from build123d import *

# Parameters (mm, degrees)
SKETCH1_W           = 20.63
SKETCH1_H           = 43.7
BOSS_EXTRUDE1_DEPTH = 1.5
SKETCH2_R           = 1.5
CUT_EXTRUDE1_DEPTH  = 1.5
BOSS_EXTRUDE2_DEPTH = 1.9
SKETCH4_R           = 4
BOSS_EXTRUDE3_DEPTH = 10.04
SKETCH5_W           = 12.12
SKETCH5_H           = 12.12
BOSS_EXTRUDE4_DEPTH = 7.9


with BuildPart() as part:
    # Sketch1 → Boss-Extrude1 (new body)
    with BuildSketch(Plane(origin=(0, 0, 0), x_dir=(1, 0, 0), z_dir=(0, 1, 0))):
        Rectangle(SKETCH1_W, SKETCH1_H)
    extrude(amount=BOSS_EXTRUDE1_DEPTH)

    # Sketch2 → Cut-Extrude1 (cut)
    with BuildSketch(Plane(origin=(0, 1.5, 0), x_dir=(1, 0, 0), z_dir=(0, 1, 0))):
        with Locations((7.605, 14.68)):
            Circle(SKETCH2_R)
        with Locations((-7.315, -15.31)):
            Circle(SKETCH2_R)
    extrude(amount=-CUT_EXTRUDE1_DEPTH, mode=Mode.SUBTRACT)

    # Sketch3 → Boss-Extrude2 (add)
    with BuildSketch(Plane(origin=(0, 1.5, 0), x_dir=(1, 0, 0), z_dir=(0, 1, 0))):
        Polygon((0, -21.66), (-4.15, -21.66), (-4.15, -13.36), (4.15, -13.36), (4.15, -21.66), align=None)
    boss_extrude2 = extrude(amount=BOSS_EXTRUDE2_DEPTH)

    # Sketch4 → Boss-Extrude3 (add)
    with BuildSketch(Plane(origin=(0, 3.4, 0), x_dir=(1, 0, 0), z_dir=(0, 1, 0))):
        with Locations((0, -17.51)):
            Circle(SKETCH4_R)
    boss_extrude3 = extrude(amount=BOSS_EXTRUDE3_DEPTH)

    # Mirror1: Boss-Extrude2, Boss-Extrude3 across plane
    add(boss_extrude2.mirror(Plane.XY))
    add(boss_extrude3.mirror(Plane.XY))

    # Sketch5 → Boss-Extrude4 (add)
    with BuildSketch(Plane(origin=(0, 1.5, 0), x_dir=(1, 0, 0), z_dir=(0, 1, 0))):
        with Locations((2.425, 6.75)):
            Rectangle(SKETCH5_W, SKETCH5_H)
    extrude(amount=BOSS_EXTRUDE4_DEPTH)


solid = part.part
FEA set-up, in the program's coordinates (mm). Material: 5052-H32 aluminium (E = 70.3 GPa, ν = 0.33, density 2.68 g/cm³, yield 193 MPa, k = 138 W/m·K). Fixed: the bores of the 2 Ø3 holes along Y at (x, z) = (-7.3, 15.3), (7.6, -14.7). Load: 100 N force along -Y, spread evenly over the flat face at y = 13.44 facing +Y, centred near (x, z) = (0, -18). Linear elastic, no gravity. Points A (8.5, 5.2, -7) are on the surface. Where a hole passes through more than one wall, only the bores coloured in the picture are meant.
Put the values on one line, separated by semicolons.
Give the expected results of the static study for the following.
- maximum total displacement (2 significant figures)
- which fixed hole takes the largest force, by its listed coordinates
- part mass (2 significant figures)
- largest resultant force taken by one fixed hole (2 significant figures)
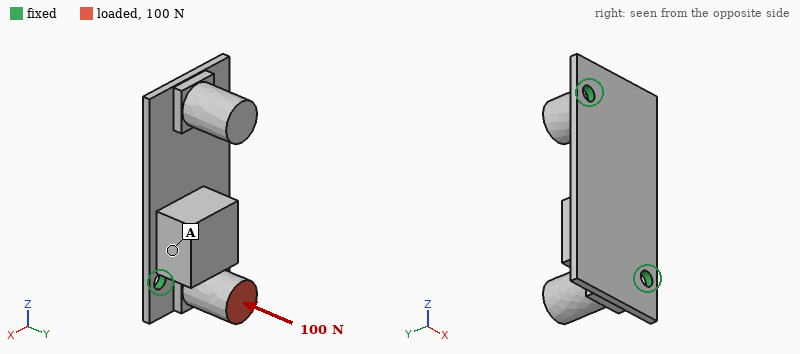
62 µm; (7.6, -14.7); 10 g; 99 N
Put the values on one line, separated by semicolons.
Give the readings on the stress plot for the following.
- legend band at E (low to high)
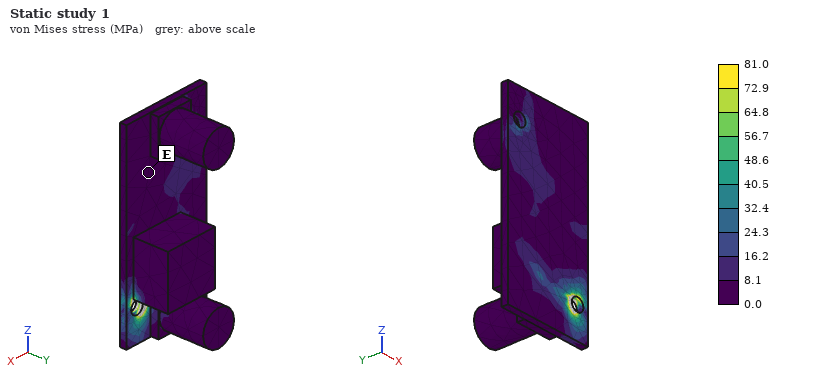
0.0 to 8.1 MPa
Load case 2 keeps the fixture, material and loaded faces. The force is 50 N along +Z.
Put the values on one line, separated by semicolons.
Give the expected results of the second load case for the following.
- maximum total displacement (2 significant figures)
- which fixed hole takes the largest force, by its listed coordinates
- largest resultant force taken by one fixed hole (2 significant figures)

46 µm; (7.6, -14.7); 32 N
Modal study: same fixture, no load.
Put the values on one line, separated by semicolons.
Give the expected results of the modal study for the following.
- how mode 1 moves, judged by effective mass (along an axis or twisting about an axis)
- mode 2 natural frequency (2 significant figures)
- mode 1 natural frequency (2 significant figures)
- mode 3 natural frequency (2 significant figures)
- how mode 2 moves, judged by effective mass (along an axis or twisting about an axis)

along X; 3900 Hz; 3300 Hz; 4900 Hz; along Y
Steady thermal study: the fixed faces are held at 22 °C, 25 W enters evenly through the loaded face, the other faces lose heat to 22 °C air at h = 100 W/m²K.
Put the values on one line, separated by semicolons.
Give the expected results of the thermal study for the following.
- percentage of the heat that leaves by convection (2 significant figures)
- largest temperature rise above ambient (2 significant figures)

20 %; 76 K
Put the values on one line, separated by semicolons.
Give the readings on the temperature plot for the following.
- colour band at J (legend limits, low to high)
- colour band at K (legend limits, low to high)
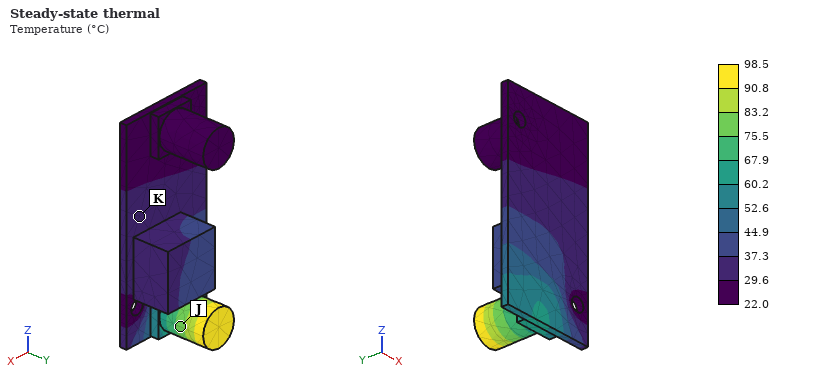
75.5 to 83.2 °C; 29.6 to 37.3 °C
